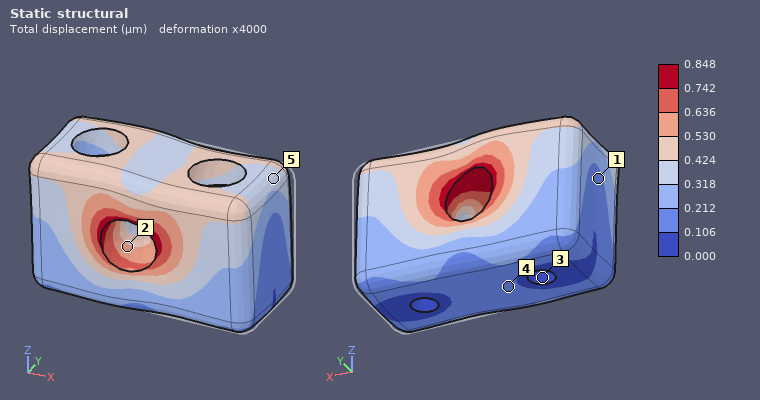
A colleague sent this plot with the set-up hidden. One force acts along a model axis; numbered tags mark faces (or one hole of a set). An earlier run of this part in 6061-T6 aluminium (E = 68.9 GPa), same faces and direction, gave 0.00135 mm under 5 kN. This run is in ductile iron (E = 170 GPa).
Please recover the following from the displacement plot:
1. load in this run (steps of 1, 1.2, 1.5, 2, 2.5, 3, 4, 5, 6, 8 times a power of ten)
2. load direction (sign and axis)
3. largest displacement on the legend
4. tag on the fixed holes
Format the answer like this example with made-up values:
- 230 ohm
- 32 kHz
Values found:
- 8 kN
- -X
- 0.848 µm
- 3
